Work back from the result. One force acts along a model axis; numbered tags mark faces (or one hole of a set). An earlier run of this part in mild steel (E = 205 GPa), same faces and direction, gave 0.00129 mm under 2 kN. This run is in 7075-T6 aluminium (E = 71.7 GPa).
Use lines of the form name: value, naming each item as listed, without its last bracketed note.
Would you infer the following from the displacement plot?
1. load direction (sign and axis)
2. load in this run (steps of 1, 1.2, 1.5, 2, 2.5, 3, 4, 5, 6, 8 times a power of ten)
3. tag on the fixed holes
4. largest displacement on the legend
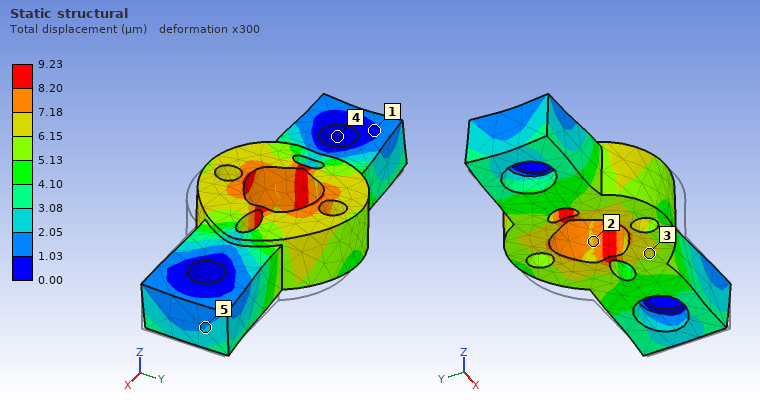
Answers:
load direction: -X
load in this run: 5 kN
tag on the fixed holes: 4
largest displacement on the legend: 9.23 µm
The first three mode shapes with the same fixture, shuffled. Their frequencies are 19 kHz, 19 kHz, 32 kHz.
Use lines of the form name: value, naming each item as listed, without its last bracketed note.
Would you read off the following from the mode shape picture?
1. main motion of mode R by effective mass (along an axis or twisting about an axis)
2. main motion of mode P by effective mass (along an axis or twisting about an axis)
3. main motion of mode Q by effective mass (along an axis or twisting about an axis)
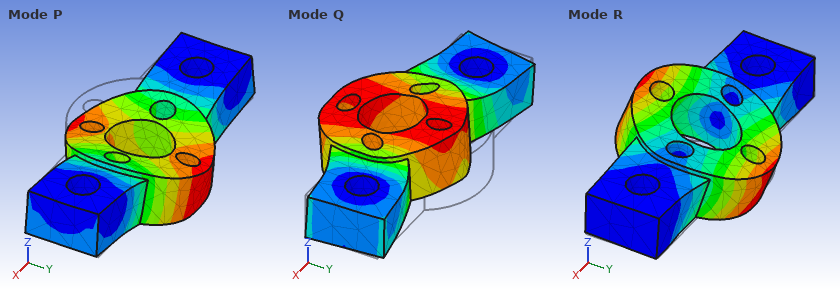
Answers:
main motion of mode R by effective mass: twisting about X
main motion of mode P by effective mass: along Z
main motion of mode Q by effective mass: along Y
